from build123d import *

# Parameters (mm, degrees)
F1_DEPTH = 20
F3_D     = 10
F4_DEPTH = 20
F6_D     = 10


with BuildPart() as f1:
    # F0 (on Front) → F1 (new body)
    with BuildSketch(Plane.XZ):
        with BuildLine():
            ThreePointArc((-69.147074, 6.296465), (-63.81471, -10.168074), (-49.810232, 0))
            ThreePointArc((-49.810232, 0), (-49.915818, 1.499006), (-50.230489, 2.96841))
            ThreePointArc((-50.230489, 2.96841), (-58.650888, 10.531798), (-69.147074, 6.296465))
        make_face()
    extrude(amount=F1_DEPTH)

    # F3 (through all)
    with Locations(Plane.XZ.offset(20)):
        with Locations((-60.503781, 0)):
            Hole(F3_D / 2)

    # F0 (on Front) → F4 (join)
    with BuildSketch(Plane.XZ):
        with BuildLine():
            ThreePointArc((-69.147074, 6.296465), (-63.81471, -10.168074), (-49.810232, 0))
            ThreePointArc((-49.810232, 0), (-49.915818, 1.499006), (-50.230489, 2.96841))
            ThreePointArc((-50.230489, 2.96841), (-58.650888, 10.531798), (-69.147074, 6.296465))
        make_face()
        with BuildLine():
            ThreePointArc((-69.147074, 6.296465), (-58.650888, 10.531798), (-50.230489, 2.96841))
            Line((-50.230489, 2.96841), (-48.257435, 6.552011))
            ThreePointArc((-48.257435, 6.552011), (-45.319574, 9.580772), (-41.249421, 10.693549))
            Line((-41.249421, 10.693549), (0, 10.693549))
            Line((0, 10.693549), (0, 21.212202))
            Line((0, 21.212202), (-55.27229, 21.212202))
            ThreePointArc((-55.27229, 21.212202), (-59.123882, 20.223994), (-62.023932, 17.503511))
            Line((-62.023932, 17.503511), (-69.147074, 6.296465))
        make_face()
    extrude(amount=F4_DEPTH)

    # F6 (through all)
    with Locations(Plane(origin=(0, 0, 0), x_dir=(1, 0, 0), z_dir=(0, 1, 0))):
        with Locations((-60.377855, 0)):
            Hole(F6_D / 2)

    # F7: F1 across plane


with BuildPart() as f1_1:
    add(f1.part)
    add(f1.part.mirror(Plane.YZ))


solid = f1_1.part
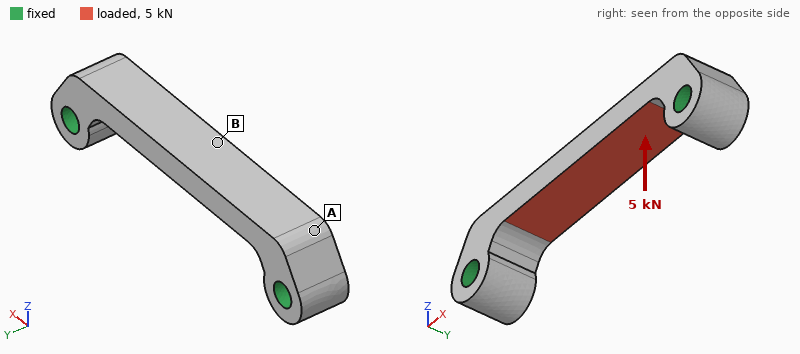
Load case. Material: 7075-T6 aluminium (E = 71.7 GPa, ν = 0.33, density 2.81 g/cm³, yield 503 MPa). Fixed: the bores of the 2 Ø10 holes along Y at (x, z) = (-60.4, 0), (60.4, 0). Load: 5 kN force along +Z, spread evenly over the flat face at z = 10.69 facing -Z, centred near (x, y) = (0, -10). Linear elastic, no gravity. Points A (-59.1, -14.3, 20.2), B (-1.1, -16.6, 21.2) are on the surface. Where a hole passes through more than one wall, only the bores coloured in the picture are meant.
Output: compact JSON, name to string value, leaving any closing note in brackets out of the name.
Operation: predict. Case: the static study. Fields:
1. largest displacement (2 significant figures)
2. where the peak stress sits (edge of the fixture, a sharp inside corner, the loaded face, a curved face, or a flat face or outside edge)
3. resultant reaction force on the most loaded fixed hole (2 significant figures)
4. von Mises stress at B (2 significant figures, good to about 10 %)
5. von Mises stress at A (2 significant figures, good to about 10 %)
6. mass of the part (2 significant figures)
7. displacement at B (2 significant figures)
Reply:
{"largest displacement": "0.15 mm", "where the peak stress sits": "a curved face", "resultant reaction force on the most loaded fixed hole": "3.6 kN", "von Mises stress at B": "84 MPa", "von Mises stress at A": "16 MPa", "mass of the part": "110 g", "displacement at B": "0.14 mm"}
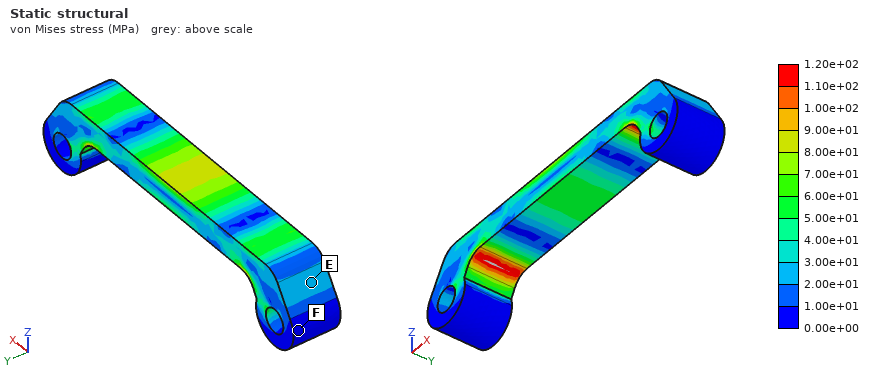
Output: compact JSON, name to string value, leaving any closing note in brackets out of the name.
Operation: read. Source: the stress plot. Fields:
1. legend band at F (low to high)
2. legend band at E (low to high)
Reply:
{"legend band at F": "0.00e+00 to 1.00e+01 MPa", "legend band at E": "2.00e+01 to 3.00e+01 MPa"}
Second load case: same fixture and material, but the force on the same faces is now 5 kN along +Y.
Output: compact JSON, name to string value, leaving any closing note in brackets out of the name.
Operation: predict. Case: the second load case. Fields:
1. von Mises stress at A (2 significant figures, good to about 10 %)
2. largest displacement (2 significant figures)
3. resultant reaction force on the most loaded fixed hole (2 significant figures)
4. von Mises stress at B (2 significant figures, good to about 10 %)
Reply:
{"von Mises stress at A": "17 MPa", "largest displacement": "0.11 mm", "resultant reaction force on the most loaded fixed hole": "2.5 kN", "von Mises stress at B": "39 MPa"}
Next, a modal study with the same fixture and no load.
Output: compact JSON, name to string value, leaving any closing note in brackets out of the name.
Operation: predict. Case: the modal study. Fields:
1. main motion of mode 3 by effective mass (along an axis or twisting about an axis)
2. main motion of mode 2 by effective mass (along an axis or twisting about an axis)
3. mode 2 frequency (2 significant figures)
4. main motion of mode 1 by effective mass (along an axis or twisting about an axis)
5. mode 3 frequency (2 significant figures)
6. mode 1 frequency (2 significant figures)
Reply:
{"main motion of mode 3 by effective mass": "along X", "main motion of mode 2 by effective mass": "along Y", "mode 2 frequency": "5900 Hz", "main motion of mode 1 by effective mass": "along Z", "mode 3 frequency": "9900 Hz", "mode 1 frequency": "4700 Hz"}
